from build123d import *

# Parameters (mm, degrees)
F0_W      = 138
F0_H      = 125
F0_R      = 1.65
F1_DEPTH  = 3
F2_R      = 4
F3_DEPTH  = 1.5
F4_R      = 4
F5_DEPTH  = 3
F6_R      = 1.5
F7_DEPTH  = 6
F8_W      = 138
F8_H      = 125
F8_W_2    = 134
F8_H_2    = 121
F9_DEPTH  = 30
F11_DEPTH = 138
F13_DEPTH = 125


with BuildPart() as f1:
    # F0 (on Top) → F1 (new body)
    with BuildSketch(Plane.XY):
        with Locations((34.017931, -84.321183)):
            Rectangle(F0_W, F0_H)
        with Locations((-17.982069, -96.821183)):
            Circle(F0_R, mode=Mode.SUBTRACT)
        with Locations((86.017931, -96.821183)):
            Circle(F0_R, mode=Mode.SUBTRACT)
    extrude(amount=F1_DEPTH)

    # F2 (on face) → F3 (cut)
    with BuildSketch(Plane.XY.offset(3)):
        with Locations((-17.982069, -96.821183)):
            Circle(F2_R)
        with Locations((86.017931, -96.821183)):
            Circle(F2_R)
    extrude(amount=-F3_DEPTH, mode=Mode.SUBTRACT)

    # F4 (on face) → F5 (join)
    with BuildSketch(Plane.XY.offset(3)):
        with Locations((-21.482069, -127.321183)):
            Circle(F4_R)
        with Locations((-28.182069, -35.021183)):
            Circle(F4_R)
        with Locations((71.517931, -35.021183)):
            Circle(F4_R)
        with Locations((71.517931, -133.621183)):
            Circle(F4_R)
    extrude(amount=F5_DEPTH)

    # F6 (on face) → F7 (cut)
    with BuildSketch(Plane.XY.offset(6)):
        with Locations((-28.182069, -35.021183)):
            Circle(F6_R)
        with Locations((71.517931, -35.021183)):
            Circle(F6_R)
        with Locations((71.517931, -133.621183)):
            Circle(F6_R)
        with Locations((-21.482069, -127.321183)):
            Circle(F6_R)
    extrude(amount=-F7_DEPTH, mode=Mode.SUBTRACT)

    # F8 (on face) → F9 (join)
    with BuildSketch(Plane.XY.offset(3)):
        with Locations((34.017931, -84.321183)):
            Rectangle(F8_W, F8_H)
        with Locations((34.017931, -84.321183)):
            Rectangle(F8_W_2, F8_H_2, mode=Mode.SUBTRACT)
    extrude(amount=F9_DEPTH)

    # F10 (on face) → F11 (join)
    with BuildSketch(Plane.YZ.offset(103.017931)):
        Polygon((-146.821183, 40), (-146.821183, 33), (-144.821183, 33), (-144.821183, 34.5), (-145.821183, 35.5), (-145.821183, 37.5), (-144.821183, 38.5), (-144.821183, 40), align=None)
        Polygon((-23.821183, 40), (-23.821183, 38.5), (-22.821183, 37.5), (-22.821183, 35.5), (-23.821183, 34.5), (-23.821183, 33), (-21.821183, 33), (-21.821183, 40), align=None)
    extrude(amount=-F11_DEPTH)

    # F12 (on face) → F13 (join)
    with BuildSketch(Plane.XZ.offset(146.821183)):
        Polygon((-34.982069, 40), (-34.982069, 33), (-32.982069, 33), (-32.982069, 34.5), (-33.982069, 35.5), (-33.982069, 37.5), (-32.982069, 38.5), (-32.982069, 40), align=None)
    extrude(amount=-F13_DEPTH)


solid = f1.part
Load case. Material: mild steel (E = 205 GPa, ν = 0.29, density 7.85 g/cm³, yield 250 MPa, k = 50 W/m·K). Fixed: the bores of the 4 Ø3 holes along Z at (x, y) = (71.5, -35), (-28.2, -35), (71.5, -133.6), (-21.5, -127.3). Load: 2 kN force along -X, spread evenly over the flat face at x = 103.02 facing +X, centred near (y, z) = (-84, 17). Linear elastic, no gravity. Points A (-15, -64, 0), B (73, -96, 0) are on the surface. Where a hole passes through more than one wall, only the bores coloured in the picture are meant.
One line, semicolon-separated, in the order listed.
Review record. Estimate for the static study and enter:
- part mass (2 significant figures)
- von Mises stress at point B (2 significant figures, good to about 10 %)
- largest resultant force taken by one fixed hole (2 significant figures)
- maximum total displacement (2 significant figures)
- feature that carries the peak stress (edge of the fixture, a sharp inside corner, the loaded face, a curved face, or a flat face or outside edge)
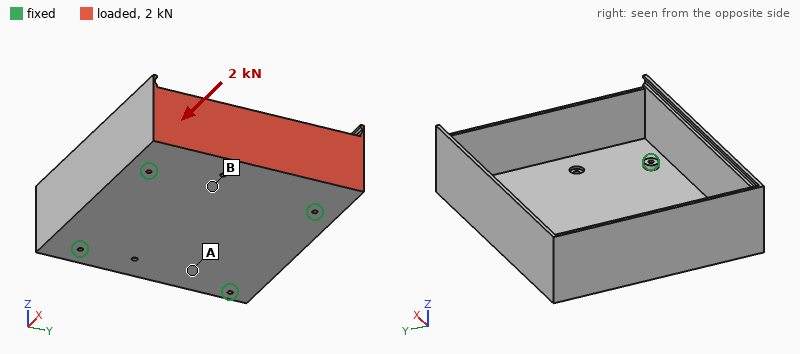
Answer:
690 g; 23 MPa; 570 N; 0.45 mm; the loaded face
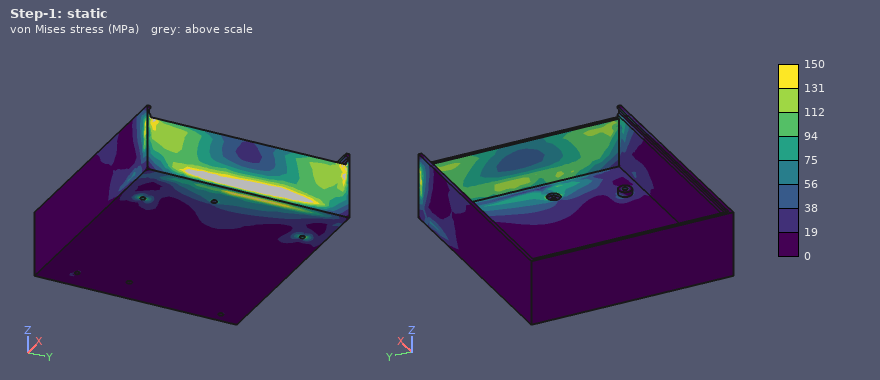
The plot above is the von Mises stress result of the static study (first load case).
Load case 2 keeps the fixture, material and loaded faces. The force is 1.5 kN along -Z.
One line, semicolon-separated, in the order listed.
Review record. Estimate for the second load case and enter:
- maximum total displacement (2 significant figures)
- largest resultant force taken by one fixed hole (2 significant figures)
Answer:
0.10 mm; 1.0 kN
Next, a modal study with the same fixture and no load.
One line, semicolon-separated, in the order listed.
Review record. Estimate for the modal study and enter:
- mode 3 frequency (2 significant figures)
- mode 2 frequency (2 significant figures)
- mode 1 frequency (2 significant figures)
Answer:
1400 Hz; 1300 Hz; 1200 Hz
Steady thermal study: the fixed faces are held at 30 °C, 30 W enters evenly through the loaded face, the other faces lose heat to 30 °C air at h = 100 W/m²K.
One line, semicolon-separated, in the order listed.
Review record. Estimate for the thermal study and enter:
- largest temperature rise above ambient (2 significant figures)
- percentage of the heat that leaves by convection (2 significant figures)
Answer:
35 K; 87 %
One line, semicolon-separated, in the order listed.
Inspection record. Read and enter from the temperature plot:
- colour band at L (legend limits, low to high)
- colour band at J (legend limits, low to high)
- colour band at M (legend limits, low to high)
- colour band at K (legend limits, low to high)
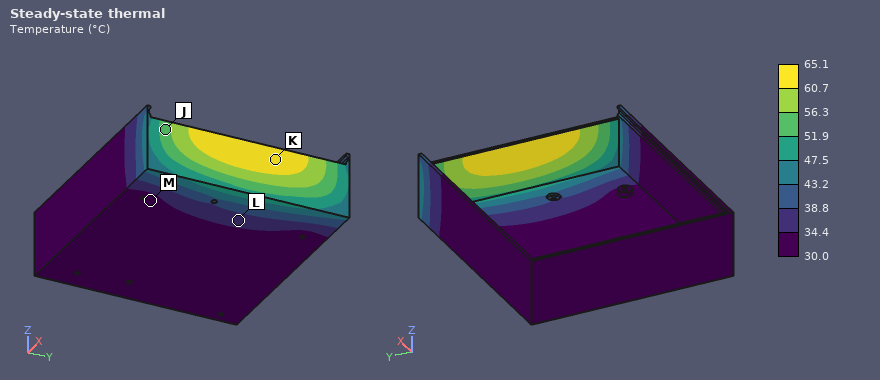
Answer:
34.4 to 38.8 °C; 51.9 to 56.3 °C; 30.0 to 34.4 °C; 60.7 to 65.1 °C
